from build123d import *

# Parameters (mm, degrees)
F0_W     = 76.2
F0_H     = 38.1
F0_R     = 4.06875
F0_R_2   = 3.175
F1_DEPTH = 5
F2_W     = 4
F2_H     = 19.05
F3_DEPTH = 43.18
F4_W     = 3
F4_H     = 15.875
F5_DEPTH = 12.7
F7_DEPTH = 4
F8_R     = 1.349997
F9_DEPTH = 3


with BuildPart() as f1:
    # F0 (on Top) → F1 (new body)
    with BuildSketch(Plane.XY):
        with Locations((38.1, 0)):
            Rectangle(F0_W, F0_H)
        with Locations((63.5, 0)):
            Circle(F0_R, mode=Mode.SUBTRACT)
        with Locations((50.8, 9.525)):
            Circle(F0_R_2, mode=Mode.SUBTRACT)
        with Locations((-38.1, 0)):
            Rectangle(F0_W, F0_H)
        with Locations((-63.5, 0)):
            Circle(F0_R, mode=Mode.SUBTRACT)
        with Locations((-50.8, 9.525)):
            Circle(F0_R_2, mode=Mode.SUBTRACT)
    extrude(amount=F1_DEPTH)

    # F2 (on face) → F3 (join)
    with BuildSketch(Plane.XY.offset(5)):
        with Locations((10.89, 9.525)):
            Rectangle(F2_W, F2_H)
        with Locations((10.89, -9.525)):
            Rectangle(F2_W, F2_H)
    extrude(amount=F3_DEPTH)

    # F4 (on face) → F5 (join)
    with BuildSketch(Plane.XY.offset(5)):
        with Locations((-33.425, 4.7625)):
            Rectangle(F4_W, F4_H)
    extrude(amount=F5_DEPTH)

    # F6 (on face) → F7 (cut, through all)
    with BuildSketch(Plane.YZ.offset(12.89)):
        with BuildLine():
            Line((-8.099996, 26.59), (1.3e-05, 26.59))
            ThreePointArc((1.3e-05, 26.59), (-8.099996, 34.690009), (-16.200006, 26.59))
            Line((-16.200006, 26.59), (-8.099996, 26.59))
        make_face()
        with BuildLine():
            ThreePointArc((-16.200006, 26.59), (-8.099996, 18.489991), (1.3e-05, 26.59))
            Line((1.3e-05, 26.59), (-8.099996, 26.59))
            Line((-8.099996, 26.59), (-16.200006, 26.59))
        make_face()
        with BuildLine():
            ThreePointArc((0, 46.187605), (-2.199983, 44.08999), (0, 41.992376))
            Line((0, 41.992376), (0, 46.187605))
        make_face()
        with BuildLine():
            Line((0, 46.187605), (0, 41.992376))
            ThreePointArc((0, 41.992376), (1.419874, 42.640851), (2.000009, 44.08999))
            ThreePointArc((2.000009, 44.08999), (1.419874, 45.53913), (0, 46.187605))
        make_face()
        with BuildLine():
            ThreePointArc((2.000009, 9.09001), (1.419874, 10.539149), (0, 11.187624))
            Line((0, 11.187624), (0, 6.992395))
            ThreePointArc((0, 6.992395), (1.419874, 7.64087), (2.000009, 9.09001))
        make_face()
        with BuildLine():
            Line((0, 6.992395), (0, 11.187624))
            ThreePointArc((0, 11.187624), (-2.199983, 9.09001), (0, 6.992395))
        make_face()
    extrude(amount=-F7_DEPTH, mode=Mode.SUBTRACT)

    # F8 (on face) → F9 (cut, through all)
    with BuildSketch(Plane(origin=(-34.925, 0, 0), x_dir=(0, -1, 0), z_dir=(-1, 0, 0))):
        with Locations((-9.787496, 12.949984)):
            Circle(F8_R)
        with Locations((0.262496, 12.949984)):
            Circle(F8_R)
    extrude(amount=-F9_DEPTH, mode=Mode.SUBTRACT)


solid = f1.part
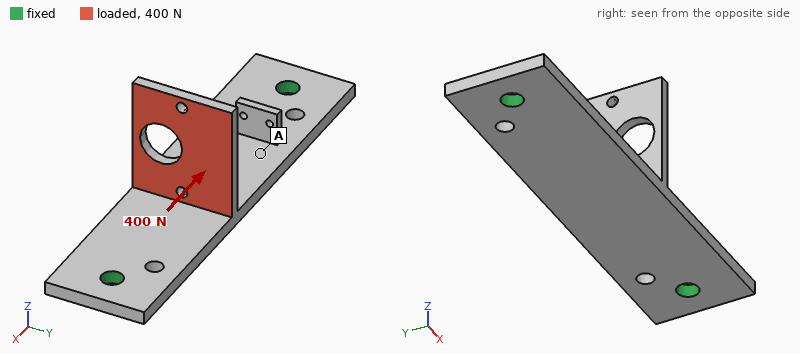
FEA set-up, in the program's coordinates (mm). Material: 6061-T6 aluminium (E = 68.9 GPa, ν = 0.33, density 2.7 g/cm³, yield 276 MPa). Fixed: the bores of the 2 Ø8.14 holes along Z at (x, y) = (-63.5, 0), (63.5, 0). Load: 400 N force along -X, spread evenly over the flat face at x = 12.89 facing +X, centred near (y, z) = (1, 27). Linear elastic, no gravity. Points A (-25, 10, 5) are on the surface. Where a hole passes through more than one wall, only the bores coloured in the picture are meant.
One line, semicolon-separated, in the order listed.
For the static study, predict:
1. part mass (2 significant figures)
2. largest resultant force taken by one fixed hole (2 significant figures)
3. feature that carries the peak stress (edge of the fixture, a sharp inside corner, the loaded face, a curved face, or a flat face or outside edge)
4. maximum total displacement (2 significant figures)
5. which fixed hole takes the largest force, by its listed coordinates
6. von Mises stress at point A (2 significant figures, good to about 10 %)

93 g; 250 N; the loaded face; 0.51 mm; (63.5, 0); 9.0 MPa
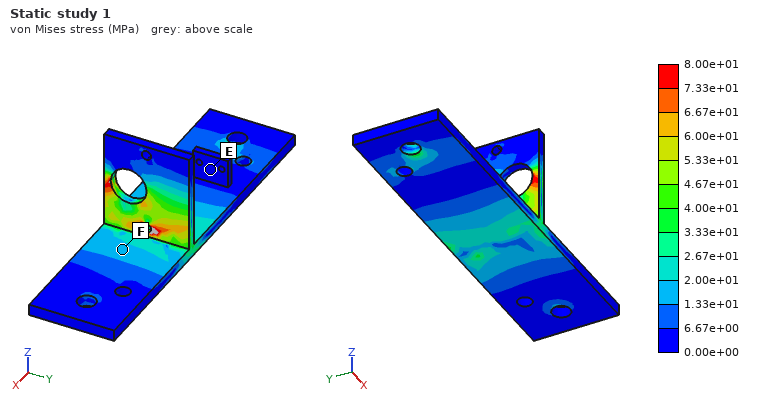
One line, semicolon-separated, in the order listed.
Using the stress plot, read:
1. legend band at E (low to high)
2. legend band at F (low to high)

0.00e+00 to 6.67e+00 MPa; 1.33e+01 to 2.00e+01 MPa
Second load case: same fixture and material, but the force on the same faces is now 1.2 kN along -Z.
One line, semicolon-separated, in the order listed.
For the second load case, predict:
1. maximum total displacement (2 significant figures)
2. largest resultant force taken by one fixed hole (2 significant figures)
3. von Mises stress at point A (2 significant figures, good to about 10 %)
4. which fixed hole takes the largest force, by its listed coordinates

0.43 mm; 780 N; 15 MPa; (63.5, 0)
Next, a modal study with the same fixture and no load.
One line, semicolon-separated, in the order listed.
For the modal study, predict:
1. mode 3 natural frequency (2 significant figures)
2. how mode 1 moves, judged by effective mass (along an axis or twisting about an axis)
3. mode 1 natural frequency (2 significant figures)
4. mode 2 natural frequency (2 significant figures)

1500 Hz; along Z; 1200 Hz; 1500 Hz
